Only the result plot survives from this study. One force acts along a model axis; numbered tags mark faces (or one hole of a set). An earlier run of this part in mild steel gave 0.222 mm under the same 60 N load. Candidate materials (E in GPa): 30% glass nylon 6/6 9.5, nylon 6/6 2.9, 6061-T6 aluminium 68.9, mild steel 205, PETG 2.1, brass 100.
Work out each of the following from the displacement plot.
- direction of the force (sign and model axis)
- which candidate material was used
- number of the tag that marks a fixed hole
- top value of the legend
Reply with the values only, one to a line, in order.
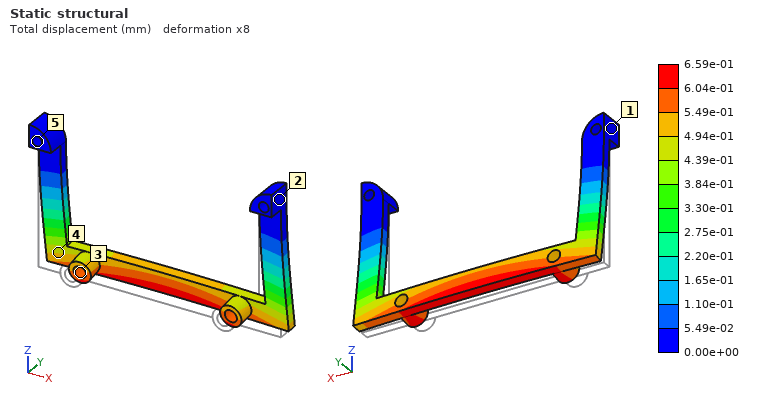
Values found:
+Y
6061-T6 aluminium
5
6.59e-01 mm
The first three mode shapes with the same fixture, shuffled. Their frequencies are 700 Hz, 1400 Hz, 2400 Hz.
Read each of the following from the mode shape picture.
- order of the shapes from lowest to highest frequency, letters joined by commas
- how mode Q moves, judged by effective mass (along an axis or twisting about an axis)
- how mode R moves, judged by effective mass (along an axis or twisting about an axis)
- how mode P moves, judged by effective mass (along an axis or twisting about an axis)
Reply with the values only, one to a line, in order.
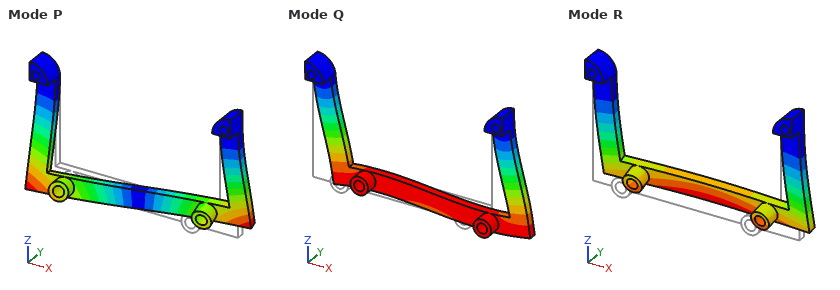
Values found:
R, P, Q
along X
along Y
twisting about Z
